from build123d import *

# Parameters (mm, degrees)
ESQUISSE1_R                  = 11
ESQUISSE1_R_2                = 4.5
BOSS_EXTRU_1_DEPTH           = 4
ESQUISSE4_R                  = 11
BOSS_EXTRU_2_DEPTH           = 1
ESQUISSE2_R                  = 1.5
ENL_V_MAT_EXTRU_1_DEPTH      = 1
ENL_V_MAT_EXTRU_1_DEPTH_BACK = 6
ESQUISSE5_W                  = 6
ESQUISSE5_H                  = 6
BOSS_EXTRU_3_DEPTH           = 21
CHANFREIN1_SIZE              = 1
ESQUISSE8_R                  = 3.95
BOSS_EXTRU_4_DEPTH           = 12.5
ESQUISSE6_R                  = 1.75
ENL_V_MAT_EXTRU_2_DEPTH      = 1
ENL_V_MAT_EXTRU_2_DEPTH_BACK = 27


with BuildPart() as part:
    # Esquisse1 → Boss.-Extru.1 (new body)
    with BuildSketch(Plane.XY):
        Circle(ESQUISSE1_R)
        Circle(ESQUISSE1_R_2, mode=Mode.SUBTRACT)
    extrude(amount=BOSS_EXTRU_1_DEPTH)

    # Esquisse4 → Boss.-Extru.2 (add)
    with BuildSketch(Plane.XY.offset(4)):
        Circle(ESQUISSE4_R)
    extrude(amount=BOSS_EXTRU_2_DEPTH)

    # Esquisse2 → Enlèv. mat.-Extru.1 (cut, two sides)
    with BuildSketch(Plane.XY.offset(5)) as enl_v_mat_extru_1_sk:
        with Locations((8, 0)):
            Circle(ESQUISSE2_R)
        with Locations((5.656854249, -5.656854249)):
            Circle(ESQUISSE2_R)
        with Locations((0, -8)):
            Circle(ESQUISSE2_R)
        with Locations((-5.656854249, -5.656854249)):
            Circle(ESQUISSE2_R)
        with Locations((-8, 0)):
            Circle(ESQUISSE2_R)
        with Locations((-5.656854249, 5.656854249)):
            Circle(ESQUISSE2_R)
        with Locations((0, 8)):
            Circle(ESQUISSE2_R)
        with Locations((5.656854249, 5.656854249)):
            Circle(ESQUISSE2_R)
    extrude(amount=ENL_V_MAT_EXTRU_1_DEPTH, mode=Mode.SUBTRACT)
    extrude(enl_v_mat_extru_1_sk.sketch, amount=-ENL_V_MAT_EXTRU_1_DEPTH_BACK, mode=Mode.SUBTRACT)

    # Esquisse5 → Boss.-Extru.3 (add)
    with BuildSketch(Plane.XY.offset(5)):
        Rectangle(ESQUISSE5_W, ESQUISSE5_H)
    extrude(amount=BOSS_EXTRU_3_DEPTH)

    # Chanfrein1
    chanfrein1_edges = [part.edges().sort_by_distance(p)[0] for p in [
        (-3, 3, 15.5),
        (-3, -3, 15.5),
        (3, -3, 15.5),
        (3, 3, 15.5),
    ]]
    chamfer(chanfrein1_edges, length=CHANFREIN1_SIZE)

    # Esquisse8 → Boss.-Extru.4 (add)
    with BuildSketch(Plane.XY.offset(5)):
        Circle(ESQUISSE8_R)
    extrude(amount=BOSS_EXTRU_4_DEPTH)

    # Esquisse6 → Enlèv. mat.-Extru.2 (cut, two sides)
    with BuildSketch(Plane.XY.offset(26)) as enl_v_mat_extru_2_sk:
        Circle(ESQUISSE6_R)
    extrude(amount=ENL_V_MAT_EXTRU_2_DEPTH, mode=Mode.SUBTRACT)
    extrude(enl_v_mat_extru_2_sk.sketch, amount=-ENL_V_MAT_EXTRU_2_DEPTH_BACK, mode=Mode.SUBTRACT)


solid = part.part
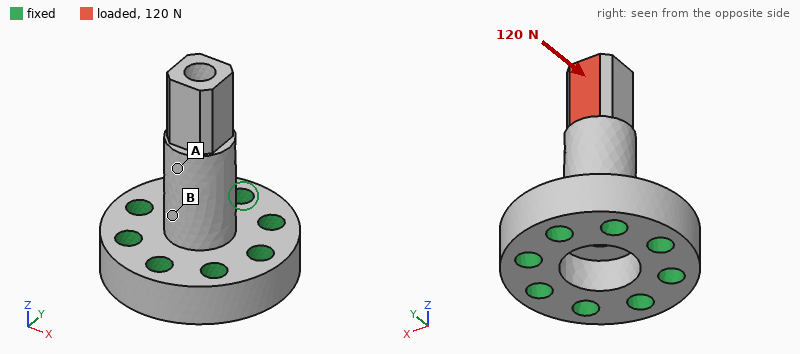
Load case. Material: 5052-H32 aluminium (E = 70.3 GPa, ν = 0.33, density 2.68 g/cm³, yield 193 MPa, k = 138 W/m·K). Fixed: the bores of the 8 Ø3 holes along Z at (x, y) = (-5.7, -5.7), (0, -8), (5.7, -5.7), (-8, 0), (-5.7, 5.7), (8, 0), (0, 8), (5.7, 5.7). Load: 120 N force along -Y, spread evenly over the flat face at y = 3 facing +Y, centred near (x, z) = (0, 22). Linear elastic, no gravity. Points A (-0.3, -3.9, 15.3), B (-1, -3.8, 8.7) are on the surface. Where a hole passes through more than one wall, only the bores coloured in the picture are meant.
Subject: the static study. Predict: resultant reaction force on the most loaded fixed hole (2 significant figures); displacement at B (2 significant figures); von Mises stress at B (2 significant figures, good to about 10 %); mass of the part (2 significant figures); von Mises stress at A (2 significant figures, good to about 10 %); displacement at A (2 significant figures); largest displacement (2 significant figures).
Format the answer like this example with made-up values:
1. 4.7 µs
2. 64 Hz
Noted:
1. 120 N
2. 7.2 µm
3. 32 MPa
4. 5.5 g
5. 14 MPa
6. 19 µm
7. 44 µm
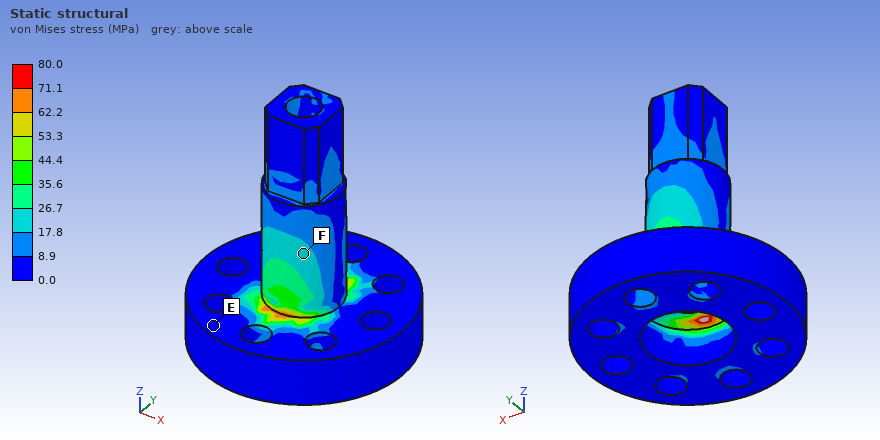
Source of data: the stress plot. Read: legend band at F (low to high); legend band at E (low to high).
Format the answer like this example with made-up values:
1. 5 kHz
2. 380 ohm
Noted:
1. 17.8 to 26.7 MPa
2. 0.0 to 8.9 MPa
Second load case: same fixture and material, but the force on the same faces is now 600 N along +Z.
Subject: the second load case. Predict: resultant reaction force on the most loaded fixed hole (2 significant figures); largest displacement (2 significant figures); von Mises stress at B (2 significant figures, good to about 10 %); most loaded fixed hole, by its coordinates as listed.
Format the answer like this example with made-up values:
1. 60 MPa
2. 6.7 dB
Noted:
1. 190 N
2. 56 µm
3. 23 MPa
4. (0, 8)
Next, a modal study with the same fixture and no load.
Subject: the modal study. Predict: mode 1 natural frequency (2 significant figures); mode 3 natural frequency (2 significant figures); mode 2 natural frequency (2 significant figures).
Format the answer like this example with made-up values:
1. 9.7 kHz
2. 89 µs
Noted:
1. 11 kHz
2. 42 kHz
3. 11 kHz
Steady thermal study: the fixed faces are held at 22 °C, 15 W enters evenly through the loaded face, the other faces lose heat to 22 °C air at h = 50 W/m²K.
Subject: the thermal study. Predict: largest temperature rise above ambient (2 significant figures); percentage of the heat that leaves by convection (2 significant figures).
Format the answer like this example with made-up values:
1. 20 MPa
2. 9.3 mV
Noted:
1. 68 K
2. 8.8 %
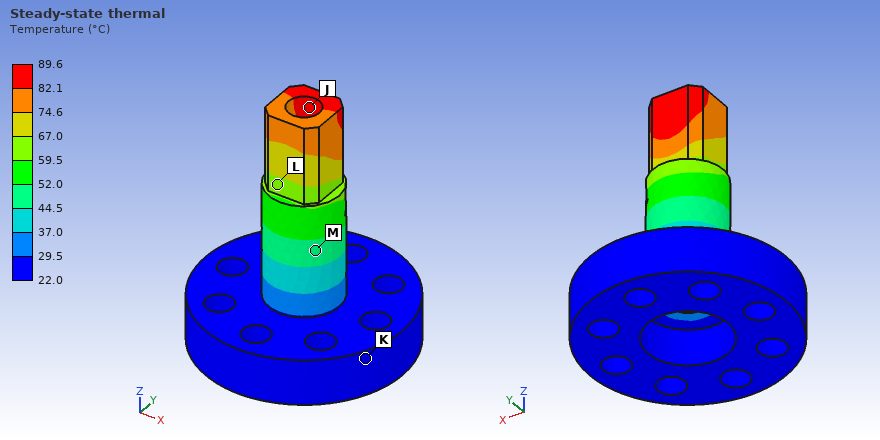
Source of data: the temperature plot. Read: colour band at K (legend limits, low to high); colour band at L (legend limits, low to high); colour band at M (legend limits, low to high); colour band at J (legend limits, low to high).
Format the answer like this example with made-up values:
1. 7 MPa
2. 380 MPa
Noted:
1. 22.0 to 29.5 °C
2. 59.5 to 67.0 °C
3. 44.5 to 52.0 °C
4. 82.1 to 89.6 °C
